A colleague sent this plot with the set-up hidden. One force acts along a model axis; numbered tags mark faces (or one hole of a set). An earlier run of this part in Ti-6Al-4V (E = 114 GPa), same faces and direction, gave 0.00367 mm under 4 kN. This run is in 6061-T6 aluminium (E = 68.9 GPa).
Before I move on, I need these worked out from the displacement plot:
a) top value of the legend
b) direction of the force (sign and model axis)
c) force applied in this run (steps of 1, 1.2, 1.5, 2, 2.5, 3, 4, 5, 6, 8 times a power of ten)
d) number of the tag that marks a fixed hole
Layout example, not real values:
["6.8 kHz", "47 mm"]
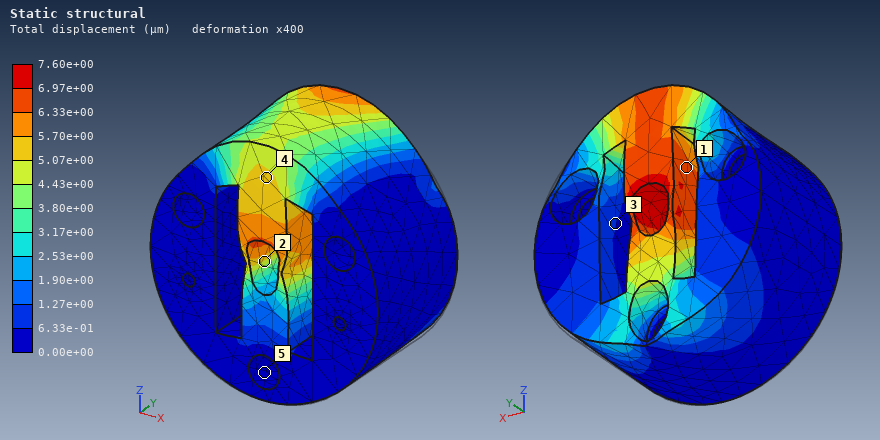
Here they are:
["7.60e+00 µm", "+Z", "5 kN", "5"]
